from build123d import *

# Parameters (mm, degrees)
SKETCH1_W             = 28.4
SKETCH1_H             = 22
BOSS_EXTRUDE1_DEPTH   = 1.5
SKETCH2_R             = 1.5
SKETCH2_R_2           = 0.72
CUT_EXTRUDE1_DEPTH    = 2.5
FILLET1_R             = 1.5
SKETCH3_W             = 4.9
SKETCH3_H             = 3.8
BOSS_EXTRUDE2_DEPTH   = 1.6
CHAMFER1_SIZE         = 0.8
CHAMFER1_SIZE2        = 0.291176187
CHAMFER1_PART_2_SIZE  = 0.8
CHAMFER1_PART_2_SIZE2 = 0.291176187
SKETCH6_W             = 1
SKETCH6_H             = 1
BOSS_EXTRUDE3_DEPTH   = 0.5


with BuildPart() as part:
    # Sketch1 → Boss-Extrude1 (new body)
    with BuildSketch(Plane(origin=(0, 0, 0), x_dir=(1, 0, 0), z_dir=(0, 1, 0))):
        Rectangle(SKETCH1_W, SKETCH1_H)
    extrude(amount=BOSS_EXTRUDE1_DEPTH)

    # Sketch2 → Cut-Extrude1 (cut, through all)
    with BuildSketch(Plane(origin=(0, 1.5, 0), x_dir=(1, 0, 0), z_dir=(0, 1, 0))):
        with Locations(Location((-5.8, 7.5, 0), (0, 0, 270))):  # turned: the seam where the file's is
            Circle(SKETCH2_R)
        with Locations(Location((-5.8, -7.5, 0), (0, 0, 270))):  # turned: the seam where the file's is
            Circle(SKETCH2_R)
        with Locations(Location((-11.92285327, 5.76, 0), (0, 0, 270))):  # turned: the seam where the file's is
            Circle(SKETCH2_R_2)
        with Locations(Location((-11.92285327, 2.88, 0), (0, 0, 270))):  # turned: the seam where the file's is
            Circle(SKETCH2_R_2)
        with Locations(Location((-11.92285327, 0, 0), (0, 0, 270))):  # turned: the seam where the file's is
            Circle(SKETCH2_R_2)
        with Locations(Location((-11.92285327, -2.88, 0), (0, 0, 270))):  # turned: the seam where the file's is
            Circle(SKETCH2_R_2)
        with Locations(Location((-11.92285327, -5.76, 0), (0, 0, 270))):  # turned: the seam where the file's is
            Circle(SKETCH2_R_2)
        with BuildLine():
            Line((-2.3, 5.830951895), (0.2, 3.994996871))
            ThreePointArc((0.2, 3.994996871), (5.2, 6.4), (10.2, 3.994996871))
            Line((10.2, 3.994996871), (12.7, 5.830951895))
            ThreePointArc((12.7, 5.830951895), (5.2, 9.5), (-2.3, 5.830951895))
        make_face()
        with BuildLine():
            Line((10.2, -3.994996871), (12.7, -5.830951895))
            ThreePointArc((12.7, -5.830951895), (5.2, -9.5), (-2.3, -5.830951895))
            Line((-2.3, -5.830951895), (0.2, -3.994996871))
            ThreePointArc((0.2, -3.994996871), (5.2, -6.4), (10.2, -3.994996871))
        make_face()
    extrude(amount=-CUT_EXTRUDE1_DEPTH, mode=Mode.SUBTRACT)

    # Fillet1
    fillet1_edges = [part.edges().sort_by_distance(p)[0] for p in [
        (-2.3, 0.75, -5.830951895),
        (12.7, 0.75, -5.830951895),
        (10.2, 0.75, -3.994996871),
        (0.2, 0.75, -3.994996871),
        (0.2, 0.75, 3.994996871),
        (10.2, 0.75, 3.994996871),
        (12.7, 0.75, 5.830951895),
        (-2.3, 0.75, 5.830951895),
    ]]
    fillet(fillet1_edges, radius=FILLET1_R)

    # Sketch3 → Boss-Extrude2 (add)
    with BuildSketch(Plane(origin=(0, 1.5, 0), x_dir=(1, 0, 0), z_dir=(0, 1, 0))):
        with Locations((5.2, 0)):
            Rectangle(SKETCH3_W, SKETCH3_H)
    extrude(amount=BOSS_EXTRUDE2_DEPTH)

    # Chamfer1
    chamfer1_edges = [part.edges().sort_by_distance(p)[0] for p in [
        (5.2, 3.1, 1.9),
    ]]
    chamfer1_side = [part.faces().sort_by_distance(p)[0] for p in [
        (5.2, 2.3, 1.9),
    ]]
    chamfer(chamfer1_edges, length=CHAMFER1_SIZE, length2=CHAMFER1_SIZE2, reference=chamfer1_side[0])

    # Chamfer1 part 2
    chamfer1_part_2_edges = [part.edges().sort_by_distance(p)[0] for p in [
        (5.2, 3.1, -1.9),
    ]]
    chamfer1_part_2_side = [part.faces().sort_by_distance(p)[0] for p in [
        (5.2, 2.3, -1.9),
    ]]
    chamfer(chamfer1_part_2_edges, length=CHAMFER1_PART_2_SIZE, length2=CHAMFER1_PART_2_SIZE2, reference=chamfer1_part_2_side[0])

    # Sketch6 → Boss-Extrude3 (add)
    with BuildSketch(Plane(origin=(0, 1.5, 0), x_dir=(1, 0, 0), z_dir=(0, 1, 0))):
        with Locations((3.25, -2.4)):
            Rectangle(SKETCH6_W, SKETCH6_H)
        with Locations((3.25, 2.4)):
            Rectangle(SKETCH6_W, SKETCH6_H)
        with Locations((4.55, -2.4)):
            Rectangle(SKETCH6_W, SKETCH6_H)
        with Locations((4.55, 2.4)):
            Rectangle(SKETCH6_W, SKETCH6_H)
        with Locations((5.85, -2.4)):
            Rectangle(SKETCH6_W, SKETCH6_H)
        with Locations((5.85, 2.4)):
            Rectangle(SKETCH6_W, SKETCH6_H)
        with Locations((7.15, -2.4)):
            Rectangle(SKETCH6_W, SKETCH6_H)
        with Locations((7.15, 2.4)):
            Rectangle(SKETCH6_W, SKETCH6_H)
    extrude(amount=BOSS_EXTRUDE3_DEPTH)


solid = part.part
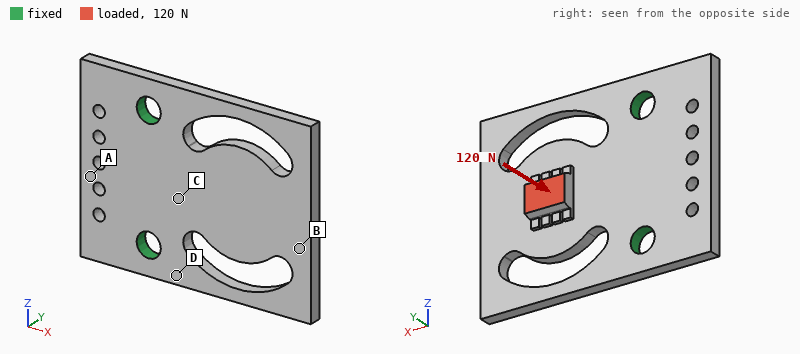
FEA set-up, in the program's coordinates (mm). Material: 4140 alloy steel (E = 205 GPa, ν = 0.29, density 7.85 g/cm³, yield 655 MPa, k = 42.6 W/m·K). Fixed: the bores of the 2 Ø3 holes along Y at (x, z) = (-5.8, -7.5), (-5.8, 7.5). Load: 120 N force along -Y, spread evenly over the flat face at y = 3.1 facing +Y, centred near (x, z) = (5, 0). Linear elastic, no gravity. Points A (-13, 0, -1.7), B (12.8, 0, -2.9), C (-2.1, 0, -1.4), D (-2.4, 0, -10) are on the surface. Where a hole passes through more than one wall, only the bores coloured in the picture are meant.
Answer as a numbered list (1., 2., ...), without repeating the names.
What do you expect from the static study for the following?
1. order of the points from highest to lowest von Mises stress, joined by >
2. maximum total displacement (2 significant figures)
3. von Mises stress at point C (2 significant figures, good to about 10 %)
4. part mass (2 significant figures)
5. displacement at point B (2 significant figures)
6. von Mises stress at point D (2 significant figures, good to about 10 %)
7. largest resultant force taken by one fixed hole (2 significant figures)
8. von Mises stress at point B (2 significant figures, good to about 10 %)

1. C > D > B > A
2. 0.12 mm
3. 130 MPa
4. 6.3 g
5. 0.11 mm
6. 100 MPa
7. 60 N
8. 42 MPa
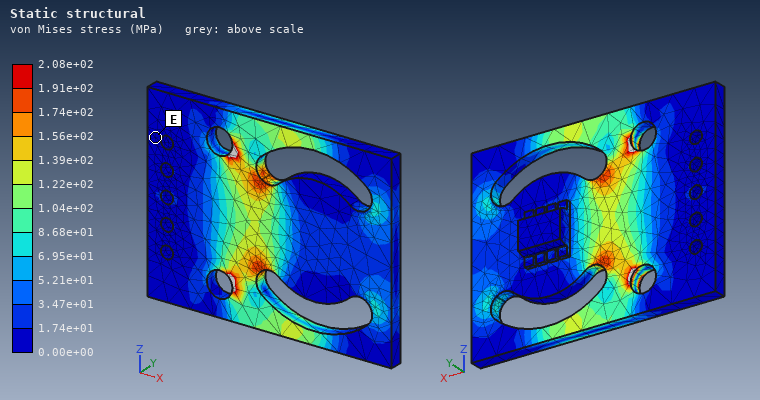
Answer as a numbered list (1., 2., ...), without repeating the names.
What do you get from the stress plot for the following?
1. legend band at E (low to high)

1. 0.00e+00 to 1.74e+01 MPa
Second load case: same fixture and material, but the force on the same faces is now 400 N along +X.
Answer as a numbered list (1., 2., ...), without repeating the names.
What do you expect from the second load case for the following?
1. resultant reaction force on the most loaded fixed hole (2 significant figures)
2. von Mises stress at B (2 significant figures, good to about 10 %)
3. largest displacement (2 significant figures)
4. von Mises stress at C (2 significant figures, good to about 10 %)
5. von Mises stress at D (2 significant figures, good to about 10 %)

1. 210 N
2. 48 MPa
3. 0.14 mm
4. 120 MPa
5. 100 MPa
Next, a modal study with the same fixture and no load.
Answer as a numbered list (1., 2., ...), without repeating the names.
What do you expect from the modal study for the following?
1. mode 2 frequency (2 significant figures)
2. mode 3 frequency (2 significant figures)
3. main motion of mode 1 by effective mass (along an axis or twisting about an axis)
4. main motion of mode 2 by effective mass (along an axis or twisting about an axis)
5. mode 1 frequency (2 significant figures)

1. 7500 Hz
2. 14 kHz
3. along Y
4. twisting about X
5. 3100 Hz
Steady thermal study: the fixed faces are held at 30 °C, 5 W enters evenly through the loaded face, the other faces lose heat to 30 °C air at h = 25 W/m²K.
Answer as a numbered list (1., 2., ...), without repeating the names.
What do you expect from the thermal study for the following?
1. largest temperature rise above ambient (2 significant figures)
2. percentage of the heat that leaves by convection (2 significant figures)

1. 74 K
2. 16 %
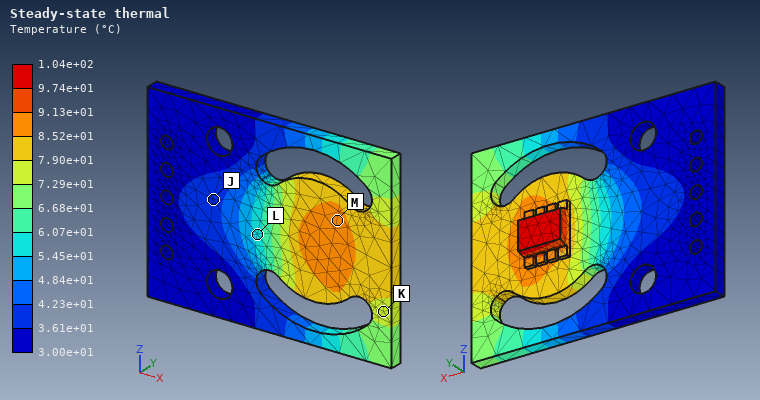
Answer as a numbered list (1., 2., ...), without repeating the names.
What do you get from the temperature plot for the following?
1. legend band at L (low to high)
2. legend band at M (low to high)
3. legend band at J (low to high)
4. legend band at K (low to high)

1. 5.45e+01 to 6.07e+01 °C
2. 8.52e+01 to 9.13e+01 °C
3. 3.61e+01 to 4.23e+01 °C
4. 7.29e+01 to 7.90e+01 °C
